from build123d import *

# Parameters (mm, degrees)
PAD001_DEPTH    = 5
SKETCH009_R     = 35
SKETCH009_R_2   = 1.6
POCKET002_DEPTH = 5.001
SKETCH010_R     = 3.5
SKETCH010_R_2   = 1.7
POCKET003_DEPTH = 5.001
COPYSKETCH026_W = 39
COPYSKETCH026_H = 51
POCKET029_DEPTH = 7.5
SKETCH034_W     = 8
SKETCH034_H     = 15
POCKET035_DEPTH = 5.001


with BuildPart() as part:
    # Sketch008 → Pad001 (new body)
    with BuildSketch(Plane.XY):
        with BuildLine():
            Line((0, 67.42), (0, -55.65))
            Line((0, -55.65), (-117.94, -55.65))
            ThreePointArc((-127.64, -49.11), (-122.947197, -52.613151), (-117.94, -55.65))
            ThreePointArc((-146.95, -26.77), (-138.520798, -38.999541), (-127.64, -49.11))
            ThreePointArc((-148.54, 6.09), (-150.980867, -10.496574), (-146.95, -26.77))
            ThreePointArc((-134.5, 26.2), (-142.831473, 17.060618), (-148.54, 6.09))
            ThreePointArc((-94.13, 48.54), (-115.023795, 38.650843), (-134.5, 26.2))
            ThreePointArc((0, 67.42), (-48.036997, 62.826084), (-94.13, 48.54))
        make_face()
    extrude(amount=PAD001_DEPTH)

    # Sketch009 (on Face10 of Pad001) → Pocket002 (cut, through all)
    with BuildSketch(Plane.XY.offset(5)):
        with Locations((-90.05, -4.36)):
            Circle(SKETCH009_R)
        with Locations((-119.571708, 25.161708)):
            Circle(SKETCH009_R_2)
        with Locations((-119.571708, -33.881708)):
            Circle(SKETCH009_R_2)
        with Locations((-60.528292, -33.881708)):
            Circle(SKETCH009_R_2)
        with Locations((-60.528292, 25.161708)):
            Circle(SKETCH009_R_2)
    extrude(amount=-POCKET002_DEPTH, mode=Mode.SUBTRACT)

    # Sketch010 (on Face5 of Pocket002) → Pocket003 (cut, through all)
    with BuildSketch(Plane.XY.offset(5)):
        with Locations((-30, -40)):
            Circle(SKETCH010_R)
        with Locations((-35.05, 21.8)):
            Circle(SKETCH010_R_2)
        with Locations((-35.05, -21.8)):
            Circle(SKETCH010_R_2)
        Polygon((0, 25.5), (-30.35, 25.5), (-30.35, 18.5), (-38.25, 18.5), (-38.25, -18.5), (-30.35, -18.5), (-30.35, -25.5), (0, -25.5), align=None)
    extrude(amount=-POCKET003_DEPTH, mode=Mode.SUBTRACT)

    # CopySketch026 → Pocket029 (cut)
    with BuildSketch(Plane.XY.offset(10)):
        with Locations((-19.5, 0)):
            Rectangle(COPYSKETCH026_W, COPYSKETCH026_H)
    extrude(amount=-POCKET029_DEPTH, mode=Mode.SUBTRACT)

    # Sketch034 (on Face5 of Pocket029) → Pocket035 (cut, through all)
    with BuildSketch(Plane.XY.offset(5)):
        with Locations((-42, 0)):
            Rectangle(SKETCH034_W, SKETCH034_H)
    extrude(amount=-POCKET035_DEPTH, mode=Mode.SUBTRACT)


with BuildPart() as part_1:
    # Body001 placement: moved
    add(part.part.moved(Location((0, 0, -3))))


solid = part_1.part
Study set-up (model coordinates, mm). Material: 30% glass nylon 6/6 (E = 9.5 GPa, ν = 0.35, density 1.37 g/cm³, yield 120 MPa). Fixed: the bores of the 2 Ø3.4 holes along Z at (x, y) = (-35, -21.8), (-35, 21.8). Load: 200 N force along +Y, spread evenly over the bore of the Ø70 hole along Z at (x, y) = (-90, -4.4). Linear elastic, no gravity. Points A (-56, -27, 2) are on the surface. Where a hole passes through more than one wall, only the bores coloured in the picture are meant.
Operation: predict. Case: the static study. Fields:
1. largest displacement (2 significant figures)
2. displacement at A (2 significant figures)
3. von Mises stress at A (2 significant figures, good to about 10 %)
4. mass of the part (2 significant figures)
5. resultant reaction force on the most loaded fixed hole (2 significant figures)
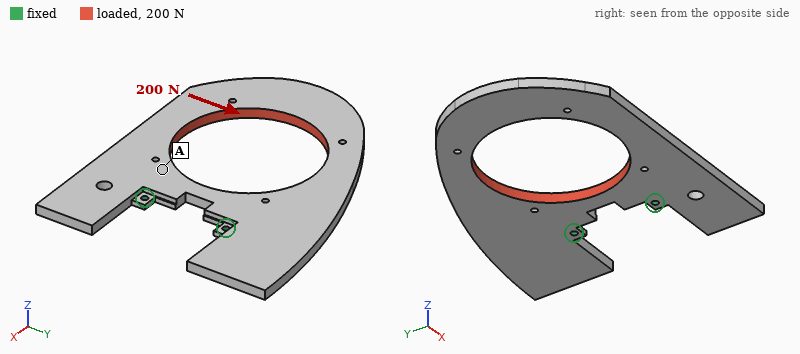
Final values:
0.29 mm
0.062 mm
2.8 MPa
65 g
240 N
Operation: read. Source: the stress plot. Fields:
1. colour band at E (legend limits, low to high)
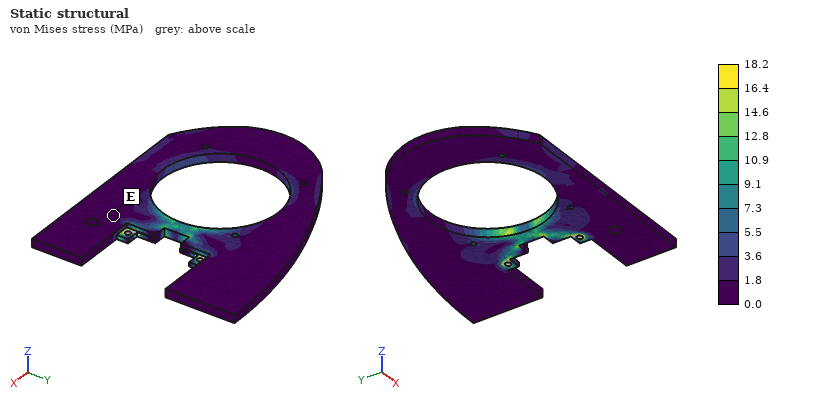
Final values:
0.0 to 1.8 MPa
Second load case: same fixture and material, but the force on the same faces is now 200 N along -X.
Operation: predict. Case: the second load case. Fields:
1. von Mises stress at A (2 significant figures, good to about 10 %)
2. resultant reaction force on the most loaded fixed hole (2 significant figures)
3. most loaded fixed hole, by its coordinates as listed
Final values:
1.2 MPa
120 N
(-35, -21.8)
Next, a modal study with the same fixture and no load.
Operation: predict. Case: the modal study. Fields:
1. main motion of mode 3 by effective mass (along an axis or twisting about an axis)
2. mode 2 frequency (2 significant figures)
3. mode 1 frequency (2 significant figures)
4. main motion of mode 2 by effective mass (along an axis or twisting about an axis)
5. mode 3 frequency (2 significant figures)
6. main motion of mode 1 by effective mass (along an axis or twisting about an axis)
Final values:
along Z
310 Hz
110 Hz
twisting about X
500 Hz
along Z
